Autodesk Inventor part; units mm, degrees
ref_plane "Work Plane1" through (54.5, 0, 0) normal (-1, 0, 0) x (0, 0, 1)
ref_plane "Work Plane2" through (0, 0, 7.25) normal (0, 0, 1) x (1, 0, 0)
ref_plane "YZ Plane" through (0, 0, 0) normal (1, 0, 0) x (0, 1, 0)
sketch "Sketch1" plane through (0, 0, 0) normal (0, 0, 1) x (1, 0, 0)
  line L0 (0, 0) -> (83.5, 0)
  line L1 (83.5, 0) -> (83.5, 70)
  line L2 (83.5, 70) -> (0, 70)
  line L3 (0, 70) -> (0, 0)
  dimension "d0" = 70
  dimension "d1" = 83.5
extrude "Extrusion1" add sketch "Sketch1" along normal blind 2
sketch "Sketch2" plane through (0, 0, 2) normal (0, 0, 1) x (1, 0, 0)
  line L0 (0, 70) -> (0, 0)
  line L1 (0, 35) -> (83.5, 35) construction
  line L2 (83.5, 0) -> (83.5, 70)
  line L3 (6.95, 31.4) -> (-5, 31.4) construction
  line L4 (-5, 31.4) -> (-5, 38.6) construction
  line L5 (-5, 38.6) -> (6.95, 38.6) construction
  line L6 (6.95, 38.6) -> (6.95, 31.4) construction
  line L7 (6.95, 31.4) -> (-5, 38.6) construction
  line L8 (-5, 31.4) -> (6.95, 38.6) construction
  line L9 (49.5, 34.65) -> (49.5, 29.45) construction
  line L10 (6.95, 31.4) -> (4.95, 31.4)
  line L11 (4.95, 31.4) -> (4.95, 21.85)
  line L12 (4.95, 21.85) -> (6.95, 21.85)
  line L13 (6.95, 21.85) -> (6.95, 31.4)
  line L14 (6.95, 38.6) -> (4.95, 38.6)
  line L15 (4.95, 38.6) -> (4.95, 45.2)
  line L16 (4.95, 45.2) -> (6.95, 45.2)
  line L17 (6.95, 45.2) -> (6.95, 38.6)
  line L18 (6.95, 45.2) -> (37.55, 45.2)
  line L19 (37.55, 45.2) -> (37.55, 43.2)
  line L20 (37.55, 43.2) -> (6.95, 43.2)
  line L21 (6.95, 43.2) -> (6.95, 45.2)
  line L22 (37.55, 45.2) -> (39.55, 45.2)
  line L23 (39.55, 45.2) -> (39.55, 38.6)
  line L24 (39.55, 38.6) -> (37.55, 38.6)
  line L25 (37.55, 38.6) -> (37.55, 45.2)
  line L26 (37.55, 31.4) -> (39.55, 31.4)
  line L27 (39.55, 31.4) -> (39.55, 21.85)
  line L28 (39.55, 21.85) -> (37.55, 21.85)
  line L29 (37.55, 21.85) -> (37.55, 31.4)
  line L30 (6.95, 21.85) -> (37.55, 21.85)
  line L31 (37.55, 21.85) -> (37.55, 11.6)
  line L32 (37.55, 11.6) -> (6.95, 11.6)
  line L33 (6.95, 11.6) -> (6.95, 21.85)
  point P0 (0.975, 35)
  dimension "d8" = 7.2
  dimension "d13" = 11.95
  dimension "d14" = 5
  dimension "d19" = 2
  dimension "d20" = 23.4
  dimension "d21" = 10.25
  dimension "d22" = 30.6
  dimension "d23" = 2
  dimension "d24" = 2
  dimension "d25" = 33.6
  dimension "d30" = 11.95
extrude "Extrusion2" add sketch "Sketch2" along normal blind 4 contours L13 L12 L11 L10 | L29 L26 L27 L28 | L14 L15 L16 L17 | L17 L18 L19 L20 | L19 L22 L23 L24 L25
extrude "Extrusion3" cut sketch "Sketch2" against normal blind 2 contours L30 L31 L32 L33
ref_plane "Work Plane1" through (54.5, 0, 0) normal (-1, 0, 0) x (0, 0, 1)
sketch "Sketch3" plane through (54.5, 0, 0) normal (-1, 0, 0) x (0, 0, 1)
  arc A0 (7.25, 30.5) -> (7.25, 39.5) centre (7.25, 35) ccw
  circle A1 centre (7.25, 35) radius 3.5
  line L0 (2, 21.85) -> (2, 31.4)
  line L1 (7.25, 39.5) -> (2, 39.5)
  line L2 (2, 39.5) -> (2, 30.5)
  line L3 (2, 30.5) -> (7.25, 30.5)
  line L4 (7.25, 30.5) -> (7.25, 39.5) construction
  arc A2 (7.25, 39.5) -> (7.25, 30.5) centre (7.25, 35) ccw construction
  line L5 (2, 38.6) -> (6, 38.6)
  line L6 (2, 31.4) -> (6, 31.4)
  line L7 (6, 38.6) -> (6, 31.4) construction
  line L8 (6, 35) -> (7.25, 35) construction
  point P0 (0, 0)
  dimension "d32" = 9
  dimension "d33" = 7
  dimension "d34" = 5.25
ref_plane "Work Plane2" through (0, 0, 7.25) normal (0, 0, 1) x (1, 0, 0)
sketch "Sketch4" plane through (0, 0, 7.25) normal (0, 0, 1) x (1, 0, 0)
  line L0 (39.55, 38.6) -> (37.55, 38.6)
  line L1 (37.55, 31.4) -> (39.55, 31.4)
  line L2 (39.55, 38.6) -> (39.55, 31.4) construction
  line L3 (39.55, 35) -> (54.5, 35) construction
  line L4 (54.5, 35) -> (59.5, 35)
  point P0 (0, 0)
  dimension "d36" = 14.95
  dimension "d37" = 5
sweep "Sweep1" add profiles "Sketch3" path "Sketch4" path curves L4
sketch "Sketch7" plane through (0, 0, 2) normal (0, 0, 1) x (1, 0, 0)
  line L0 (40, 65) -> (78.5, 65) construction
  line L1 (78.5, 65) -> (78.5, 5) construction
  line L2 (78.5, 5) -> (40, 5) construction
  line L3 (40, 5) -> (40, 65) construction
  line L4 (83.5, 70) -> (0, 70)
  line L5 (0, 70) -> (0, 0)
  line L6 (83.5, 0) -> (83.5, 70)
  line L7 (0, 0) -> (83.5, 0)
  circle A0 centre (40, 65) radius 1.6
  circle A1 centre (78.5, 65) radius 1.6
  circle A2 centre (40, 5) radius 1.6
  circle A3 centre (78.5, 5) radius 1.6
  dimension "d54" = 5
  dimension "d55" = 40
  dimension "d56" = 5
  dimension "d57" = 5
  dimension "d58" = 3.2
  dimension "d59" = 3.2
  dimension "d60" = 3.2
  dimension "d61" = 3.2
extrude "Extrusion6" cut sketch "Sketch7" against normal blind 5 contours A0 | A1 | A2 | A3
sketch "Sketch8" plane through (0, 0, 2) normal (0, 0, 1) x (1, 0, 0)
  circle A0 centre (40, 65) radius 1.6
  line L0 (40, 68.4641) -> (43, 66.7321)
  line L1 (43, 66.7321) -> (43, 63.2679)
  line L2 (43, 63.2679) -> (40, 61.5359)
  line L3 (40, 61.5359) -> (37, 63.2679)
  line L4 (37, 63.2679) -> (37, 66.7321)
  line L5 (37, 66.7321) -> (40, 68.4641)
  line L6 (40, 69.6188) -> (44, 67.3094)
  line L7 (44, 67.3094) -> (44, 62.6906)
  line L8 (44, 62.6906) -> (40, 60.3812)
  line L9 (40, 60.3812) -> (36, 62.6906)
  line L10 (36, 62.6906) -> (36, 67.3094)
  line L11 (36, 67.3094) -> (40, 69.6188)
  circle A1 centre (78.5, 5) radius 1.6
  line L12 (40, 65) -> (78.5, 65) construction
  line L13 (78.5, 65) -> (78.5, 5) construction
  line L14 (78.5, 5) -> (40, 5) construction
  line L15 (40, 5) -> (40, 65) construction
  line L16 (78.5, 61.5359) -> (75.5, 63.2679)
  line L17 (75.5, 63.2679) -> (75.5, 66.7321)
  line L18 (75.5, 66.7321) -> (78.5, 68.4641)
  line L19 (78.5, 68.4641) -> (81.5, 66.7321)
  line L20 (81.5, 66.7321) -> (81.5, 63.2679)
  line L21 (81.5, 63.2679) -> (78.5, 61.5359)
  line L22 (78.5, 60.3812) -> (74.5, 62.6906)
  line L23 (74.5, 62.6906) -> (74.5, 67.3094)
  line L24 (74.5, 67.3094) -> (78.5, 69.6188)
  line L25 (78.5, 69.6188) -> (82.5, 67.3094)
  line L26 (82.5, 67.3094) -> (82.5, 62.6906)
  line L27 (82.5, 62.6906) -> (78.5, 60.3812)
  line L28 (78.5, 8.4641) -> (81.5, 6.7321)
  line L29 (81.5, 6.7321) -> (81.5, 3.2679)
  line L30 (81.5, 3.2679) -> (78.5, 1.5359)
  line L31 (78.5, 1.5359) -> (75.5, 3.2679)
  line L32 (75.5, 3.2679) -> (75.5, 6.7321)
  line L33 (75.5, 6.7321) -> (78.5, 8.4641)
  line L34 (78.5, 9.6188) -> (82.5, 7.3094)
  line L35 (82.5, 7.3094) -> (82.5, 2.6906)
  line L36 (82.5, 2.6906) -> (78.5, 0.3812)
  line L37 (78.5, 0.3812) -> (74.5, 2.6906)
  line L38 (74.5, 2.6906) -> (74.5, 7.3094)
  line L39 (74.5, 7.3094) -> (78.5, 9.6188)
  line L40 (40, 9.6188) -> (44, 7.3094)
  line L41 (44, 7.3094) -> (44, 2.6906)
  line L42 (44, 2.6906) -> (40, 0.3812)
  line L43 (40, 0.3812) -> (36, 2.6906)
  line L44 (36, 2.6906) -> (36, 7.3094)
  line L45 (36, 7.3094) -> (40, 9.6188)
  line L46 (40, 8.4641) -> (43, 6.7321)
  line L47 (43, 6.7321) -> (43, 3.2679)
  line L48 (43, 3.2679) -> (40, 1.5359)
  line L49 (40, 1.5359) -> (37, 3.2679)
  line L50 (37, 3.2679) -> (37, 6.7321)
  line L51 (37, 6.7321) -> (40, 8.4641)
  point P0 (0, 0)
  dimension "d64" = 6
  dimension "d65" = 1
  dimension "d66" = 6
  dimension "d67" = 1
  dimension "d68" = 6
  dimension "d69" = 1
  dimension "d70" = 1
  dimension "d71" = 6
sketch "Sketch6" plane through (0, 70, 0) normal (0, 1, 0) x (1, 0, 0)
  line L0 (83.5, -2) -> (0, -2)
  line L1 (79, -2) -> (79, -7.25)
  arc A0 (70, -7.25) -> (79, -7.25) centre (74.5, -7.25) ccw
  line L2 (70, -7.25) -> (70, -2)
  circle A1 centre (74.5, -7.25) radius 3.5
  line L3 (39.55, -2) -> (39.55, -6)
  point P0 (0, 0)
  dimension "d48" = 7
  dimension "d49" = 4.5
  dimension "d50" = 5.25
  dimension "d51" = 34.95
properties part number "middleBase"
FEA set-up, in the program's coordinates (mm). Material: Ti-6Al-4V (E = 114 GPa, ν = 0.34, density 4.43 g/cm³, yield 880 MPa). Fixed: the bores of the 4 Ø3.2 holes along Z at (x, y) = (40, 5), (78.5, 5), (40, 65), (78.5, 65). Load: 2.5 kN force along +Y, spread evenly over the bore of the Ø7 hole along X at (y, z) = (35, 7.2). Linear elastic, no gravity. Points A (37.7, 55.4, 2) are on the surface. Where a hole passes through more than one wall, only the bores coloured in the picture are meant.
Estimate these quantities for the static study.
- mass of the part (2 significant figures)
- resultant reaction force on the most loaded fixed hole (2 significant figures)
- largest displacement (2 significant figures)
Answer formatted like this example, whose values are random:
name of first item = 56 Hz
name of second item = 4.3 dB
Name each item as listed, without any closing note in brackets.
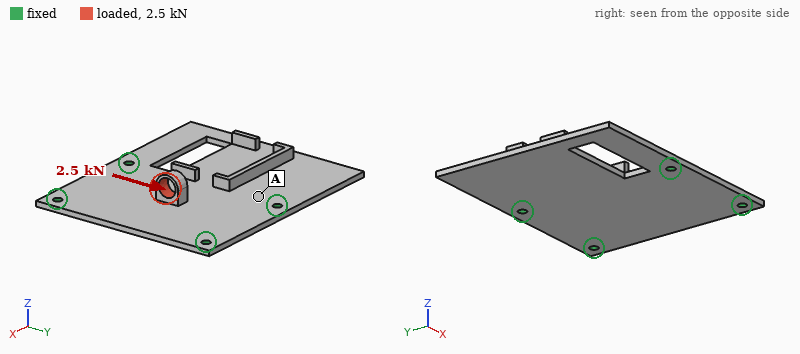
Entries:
mass of the part = 52 g
resultant reaction force on the most loaded fixed hole = 780 N
largest displacement = 0.38 mm
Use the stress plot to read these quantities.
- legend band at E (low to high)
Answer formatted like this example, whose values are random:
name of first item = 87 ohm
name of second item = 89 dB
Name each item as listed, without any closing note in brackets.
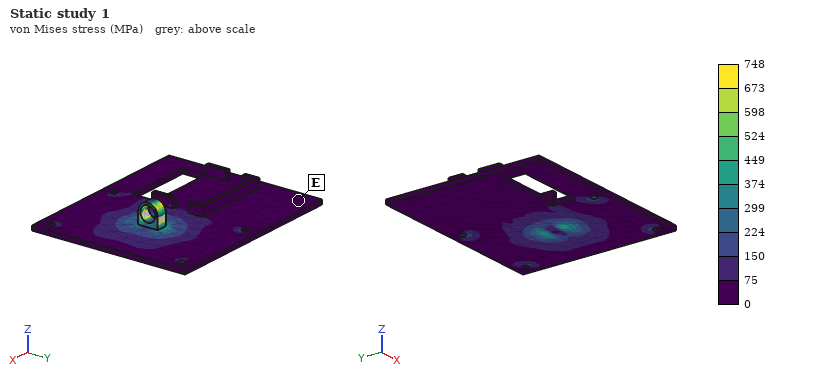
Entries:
legend band at E = 0 to 75 MPa
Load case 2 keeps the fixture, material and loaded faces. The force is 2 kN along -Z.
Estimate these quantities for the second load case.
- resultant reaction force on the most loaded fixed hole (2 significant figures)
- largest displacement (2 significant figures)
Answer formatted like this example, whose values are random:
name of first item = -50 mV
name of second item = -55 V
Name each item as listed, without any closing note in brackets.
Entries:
resultant reaction force on the most loaded fixed hole = 590 N
largest displacement = 0.75 mm
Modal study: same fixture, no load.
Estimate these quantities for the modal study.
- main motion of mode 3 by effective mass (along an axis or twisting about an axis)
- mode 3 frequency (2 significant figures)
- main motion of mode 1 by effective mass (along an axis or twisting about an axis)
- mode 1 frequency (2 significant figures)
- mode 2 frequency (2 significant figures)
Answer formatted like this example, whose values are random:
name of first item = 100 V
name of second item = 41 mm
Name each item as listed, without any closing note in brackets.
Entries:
main motion of mode 3 by effective mass = along Z
mode 3 frequency = 2400 Hz
main motion of mode 1 by effective mass = along Z
mode 1 frequency = 860 Hz
mode 2 frequency = 1700 Hz
